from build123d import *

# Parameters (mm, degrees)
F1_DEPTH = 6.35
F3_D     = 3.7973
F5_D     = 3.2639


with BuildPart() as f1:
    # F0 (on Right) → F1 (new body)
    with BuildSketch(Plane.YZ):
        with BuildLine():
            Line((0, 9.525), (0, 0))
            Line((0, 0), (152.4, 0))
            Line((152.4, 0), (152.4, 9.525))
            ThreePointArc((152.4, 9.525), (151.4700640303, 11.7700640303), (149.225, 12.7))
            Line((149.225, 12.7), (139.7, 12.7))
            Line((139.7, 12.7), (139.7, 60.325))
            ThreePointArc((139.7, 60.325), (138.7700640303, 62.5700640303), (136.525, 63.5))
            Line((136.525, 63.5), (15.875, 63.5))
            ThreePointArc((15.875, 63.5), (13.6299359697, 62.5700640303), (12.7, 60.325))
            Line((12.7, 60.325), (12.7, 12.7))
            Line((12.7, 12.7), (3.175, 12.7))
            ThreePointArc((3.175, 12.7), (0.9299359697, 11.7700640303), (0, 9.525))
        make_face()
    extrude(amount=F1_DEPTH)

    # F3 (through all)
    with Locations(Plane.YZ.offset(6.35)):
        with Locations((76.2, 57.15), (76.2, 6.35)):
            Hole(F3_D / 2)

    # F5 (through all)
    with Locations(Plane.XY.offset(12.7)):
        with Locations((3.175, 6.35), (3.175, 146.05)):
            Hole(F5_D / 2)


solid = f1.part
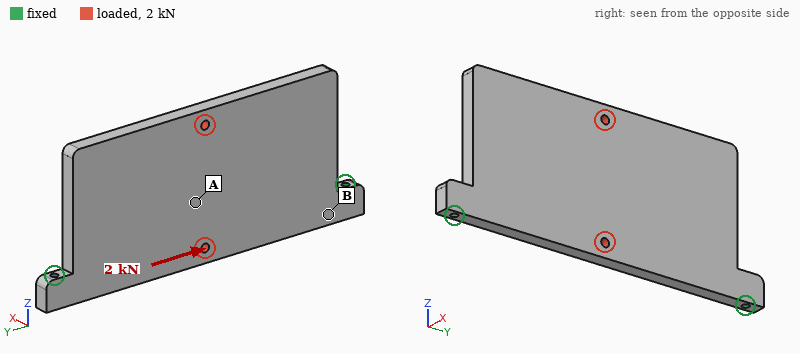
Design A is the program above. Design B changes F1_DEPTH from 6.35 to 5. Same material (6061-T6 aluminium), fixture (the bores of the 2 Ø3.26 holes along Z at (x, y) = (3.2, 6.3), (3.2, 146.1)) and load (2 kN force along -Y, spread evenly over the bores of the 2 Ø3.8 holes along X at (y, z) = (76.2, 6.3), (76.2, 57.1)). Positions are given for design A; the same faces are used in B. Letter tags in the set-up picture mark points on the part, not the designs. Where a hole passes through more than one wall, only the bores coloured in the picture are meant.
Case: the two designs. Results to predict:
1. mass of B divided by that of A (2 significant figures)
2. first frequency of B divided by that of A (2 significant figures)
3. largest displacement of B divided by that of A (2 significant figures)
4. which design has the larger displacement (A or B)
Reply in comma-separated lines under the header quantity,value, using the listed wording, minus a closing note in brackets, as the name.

quantity,value
mass of B divided by that of A,0.79
first frequency of B divided by that of A,0.82
largest displacement of B divided by that of A,1.3
which design has the larger displacement,B
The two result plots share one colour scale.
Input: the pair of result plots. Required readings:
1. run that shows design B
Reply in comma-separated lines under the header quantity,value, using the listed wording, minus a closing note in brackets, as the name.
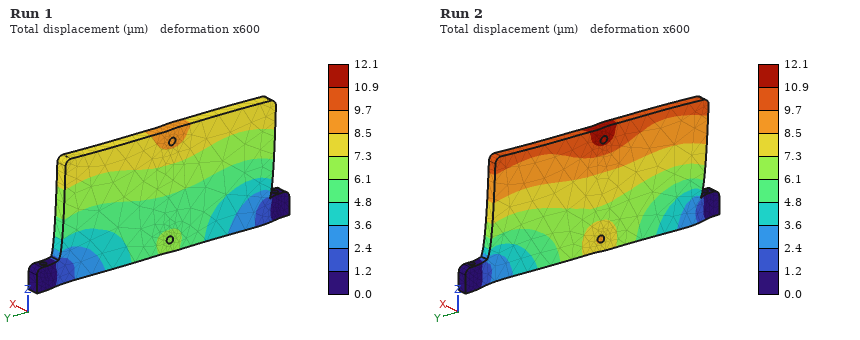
quantity,value
run that shows design B,Run 2
